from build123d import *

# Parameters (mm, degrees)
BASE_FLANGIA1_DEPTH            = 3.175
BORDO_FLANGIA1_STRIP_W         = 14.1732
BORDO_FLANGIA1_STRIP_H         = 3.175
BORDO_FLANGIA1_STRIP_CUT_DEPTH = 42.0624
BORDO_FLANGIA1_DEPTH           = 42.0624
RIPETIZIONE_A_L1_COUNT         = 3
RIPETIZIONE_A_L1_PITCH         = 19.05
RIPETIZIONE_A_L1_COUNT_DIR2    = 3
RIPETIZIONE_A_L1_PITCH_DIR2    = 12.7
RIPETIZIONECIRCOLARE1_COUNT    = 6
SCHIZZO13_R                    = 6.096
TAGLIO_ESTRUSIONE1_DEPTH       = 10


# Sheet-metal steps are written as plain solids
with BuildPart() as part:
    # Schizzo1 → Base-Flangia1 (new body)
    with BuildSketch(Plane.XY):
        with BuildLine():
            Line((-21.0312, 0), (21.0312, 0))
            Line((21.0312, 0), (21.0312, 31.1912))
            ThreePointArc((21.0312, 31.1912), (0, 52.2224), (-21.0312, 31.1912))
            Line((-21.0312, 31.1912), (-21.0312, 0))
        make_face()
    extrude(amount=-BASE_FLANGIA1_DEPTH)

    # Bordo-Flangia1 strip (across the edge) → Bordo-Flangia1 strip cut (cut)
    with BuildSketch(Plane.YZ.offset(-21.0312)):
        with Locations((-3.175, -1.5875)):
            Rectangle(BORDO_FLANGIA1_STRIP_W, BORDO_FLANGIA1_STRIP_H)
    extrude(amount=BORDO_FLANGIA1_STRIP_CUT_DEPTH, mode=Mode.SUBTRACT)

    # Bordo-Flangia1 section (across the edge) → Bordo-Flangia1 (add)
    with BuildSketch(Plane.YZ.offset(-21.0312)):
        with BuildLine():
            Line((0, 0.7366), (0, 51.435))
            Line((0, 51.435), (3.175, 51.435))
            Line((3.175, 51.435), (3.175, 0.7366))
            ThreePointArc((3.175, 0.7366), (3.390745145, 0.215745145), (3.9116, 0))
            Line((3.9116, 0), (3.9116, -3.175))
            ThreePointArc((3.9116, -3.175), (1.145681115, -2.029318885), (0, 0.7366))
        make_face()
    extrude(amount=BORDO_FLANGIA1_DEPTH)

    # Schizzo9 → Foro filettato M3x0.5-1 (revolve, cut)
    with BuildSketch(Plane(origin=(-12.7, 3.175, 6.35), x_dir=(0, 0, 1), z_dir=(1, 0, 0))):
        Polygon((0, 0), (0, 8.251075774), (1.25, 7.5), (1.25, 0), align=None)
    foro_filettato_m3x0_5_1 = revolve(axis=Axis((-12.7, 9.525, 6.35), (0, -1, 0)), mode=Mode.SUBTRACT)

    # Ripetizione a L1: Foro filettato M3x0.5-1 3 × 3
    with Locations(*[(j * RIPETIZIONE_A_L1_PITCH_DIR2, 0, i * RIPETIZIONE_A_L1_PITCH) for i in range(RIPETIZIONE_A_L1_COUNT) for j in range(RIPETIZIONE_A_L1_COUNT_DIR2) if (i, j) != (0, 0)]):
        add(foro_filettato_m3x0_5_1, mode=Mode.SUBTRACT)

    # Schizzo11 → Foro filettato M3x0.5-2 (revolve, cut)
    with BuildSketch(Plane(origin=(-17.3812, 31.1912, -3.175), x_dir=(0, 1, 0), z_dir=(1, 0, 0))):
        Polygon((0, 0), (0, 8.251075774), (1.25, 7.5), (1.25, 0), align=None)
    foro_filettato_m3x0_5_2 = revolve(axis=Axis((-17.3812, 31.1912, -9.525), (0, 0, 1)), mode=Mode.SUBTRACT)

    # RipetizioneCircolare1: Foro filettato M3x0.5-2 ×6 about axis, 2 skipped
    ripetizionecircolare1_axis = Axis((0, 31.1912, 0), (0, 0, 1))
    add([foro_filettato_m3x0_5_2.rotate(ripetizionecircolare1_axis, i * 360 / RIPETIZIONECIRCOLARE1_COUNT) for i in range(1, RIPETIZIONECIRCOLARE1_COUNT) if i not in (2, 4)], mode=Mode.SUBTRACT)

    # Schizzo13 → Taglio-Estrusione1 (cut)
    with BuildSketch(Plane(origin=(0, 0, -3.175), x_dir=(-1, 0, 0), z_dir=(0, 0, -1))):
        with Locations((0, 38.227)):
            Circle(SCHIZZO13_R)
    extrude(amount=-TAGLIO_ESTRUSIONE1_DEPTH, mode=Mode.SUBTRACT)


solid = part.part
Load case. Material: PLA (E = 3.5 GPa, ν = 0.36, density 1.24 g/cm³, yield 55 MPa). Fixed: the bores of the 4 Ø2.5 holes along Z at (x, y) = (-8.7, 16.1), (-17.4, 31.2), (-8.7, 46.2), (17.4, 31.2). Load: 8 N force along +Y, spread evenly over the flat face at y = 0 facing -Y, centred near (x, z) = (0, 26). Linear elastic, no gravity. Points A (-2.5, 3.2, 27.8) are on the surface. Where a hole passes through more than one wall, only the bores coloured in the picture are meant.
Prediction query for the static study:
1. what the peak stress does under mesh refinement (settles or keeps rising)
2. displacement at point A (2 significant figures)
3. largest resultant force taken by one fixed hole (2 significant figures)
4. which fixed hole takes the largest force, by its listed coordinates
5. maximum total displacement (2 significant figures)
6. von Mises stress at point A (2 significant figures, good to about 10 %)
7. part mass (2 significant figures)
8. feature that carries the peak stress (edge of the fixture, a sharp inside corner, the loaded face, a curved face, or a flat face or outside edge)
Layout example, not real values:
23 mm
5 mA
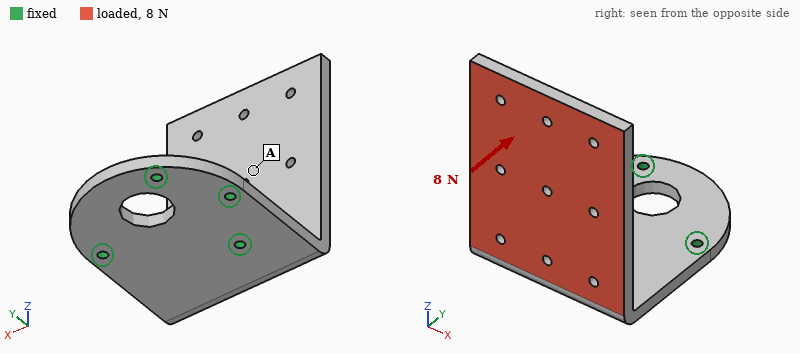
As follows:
keeps rising
0.43 mm
9.0 N
(-8.7, 16.1)
0.87 mm
0.66 MPa
16 g
edge of the fixture
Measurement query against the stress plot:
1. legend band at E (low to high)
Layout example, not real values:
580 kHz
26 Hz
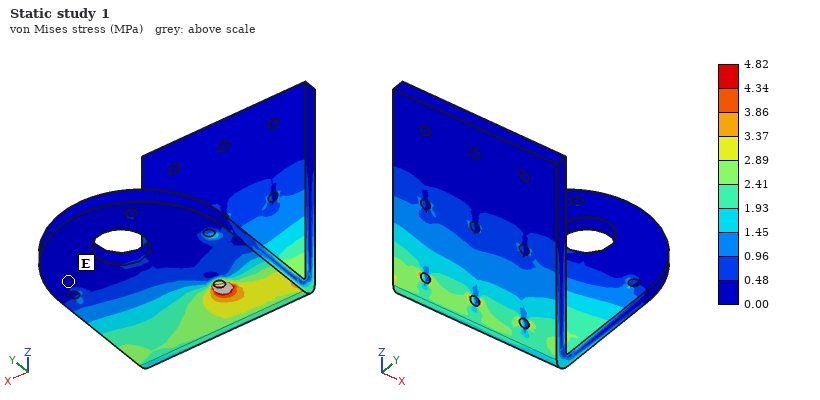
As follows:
0.00 to 0.48 MPa
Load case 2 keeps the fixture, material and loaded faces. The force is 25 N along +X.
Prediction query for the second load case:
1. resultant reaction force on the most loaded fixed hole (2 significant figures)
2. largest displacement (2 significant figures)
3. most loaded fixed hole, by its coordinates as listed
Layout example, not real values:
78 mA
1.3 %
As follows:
25 N
0.93 mm
(-8.7, 16.1)
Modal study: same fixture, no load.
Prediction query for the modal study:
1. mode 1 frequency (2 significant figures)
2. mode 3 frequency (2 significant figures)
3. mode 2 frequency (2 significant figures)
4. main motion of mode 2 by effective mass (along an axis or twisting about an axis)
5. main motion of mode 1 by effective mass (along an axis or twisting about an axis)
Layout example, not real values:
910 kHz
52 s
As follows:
200 Hz
810 Hz
350 Hz
along X
along Y
